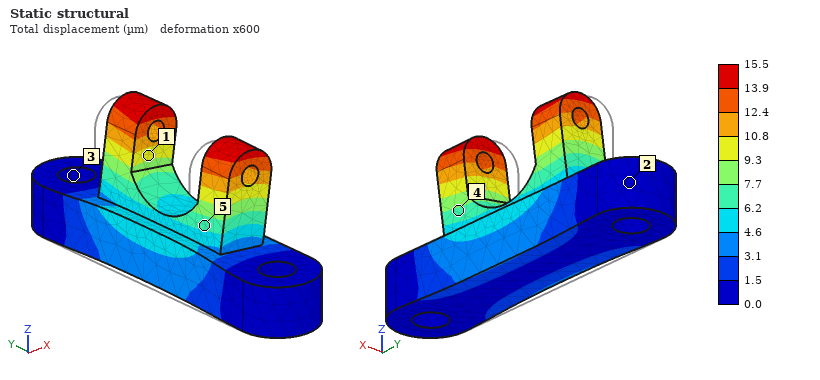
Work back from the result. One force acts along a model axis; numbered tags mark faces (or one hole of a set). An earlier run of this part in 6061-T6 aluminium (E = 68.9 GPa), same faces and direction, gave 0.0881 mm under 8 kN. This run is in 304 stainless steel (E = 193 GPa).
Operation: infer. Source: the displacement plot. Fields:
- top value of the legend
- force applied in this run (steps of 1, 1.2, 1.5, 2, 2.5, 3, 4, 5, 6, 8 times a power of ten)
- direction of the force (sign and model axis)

15.5 µm
4 kN
+X
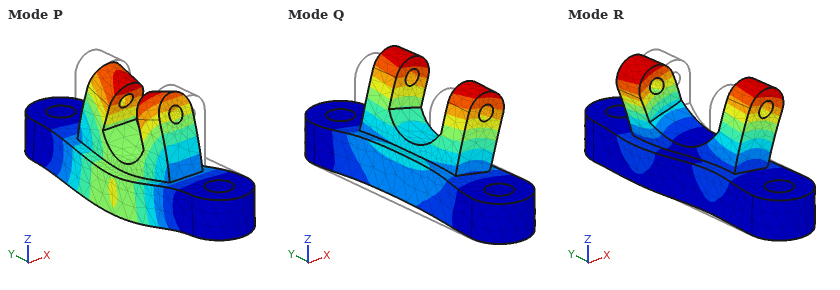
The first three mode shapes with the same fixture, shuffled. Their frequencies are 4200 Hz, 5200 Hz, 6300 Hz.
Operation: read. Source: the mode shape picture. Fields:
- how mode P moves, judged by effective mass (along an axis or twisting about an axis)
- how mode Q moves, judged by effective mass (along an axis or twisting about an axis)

along Z
along X
